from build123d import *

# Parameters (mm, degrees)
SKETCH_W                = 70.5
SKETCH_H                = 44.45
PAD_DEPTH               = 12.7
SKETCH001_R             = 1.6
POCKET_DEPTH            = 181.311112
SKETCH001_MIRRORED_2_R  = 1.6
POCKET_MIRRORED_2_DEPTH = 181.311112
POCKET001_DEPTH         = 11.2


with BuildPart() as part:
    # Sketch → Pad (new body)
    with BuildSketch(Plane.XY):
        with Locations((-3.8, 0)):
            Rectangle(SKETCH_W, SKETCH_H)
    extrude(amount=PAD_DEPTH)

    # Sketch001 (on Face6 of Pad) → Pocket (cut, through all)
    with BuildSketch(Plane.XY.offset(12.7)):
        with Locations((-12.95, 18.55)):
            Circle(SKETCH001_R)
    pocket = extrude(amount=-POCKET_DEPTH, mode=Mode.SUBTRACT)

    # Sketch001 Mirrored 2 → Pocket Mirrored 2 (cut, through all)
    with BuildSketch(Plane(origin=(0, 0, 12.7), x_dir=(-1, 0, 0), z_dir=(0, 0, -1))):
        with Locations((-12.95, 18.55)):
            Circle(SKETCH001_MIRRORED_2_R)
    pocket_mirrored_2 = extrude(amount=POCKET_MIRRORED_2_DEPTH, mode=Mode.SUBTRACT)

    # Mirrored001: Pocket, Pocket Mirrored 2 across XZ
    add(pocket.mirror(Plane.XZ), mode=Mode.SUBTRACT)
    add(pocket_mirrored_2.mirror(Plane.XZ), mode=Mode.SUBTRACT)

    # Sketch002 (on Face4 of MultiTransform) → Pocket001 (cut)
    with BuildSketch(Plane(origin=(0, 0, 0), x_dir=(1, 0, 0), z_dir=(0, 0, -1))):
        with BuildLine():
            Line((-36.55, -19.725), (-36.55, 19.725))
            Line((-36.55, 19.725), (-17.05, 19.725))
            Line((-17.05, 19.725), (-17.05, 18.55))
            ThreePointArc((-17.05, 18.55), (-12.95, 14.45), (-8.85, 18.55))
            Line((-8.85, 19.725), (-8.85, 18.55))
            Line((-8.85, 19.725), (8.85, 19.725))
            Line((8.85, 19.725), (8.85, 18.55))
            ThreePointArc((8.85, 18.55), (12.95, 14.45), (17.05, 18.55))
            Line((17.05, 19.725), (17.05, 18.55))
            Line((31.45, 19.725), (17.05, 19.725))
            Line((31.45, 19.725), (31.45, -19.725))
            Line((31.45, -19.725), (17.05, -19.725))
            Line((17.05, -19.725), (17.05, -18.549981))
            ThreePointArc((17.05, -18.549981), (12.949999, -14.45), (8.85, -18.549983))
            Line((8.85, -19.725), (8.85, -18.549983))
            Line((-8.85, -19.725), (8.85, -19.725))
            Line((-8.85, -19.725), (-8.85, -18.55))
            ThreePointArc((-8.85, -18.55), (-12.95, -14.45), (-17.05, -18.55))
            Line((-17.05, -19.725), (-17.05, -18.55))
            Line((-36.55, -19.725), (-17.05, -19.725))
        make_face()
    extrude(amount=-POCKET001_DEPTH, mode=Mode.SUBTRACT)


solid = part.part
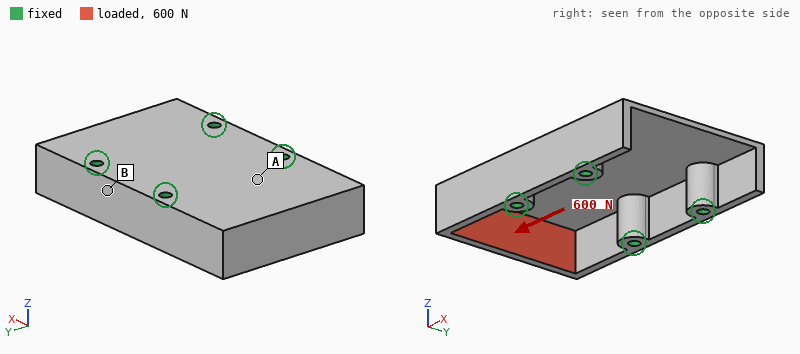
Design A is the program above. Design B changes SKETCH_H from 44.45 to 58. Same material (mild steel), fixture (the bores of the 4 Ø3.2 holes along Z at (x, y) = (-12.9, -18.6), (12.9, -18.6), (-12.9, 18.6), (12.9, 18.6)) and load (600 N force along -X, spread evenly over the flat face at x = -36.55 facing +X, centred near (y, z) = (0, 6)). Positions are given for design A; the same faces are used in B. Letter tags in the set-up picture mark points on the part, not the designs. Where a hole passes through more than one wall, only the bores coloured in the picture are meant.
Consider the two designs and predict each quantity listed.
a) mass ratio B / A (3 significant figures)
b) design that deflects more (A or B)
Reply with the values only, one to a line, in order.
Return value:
2.11
A
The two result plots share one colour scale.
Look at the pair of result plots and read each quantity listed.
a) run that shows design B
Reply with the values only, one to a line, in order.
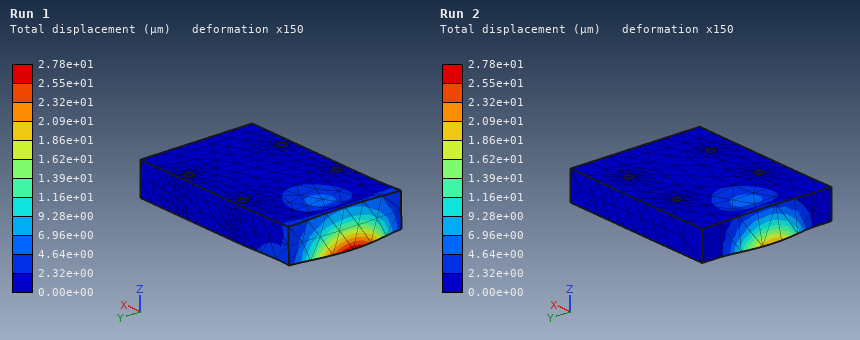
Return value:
Run 2
